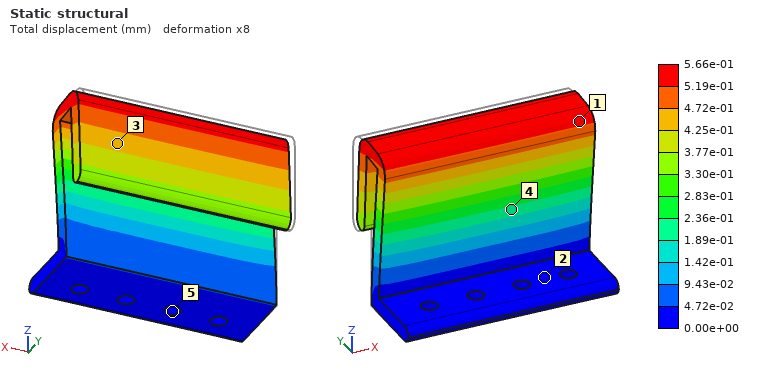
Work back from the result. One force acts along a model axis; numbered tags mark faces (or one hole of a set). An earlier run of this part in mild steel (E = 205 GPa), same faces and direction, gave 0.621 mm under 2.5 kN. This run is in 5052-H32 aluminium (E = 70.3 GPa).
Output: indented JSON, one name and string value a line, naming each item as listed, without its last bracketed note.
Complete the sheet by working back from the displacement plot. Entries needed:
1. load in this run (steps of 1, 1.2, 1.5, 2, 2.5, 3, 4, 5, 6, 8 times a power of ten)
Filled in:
{
  "load in this run": "800 N"
}
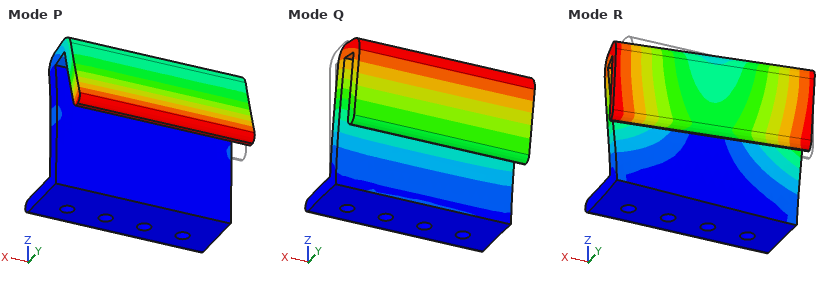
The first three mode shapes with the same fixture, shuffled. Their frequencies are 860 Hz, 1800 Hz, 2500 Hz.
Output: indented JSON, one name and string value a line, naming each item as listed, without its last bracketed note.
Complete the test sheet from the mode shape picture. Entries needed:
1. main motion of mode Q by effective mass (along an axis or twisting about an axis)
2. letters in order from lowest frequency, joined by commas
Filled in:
{
  "main motion of mode Q by effective mass": "along Y",
  "letters in order from lowest frequency, joined by commas": "Q, R, P"
}
